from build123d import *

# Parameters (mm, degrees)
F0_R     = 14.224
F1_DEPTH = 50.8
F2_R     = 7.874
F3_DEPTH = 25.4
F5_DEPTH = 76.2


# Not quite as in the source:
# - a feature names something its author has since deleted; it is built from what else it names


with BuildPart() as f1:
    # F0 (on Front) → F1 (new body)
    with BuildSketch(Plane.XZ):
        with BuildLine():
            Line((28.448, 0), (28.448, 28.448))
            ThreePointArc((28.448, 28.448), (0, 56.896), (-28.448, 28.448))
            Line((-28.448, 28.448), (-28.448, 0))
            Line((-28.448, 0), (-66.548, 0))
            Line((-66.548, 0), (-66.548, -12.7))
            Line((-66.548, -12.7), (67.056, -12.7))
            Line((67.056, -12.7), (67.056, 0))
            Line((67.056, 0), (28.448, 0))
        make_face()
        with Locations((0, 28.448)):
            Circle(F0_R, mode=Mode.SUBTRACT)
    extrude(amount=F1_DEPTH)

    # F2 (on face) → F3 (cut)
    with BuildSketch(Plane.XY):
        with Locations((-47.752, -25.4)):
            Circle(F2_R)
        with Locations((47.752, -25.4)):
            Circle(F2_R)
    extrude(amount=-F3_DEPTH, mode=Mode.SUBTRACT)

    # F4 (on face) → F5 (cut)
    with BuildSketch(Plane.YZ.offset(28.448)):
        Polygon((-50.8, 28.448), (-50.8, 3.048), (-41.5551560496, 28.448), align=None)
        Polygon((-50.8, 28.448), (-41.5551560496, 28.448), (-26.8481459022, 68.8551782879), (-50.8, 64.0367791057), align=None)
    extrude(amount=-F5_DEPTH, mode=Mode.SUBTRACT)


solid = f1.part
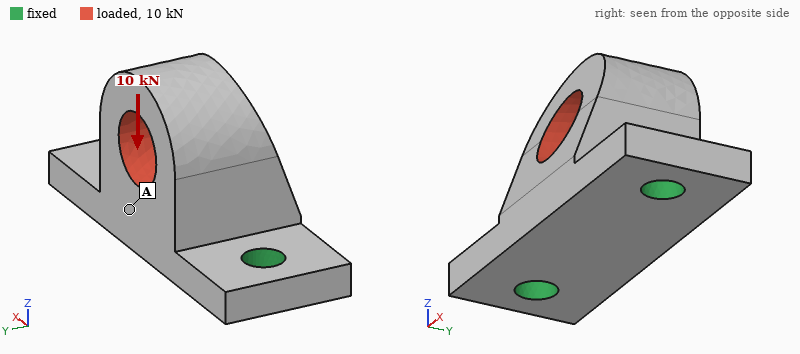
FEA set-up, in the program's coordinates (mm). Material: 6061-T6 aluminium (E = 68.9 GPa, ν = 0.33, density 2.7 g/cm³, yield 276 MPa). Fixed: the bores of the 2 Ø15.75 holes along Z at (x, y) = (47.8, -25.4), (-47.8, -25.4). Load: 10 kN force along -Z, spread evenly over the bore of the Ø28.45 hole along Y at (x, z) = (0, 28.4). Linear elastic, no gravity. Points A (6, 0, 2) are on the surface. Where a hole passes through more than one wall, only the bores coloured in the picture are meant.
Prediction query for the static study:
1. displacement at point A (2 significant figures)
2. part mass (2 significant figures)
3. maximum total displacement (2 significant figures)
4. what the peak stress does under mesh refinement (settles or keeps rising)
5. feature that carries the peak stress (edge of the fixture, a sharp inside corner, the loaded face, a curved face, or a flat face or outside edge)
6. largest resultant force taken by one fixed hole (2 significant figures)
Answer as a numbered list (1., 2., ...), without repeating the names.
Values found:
1. 30 µm
2. 480 g
3. 41 µm
4. keeps rising
5. edge of the fixture
6. 5.4 kN
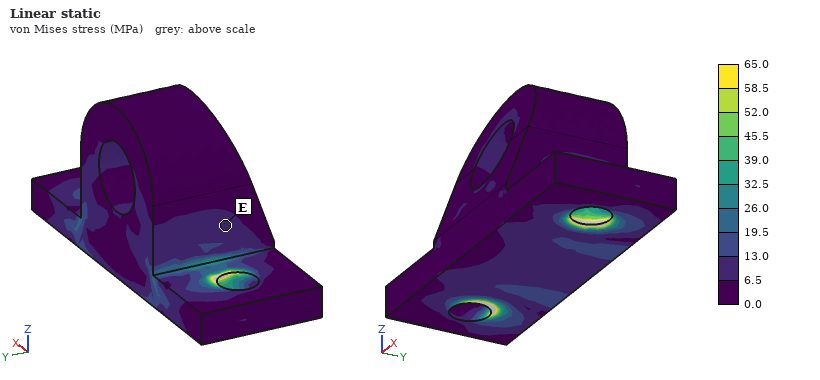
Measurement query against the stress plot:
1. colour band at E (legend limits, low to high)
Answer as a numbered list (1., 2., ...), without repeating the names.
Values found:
1. 6.5 to 13.0 MPa
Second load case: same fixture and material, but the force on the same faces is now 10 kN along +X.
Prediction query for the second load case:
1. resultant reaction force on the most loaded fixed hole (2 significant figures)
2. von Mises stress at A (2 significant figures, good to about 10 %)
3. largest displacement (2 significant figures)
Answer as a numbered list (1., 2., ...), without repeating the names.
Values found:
1. 6.9 kN
2. 8.4 MPa
3. 45 µm
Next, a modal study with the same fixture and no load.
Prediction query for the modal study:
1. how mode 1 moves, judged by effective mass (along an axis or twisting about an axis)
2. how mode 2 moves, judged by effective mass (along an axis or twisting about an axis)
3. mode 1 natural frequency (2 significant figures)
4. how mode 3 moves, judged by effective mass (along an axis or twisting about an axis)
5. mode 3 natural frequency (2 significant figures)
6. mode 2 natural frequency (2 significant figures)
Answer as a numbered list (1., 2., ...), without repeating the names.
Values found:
1. along Y
2. along X
3. 2600 Hz
4. along Z
5. 6100 Hz
6. 5700 Hz
